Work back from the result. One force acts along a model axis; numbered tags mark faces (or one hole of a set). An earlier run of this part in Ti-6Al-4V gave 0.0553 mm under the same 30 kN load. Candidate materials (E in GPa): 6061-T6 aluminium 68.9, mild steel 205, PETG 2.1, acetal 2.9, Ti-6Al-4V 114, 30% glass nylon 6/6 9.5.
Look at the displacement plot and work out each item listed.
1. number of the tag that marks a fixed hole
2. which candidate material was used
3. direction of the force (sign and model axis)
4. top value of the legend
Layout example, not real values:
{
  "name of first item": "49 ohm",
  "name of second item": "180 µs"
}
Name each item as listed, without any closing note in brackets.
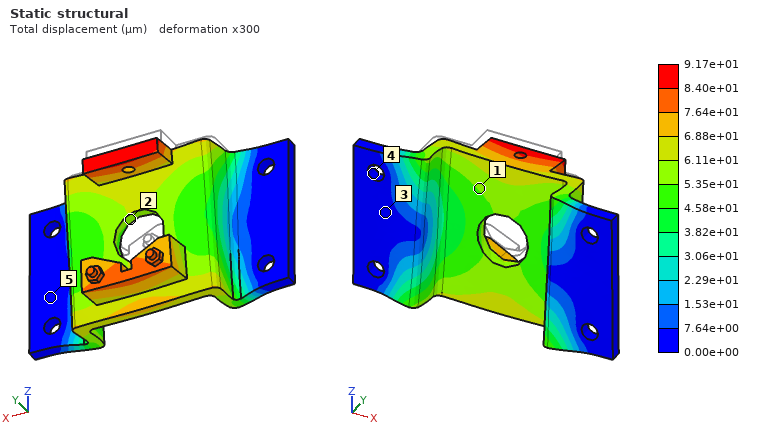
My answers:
{
  "number of the tag that marks a fixed hole": "4",
  "which candidate material was used": "6061-T6 aluminium",
  "direction of the force": "-Z",
  "top value of the legend": "9.17e+01 µm"
}
